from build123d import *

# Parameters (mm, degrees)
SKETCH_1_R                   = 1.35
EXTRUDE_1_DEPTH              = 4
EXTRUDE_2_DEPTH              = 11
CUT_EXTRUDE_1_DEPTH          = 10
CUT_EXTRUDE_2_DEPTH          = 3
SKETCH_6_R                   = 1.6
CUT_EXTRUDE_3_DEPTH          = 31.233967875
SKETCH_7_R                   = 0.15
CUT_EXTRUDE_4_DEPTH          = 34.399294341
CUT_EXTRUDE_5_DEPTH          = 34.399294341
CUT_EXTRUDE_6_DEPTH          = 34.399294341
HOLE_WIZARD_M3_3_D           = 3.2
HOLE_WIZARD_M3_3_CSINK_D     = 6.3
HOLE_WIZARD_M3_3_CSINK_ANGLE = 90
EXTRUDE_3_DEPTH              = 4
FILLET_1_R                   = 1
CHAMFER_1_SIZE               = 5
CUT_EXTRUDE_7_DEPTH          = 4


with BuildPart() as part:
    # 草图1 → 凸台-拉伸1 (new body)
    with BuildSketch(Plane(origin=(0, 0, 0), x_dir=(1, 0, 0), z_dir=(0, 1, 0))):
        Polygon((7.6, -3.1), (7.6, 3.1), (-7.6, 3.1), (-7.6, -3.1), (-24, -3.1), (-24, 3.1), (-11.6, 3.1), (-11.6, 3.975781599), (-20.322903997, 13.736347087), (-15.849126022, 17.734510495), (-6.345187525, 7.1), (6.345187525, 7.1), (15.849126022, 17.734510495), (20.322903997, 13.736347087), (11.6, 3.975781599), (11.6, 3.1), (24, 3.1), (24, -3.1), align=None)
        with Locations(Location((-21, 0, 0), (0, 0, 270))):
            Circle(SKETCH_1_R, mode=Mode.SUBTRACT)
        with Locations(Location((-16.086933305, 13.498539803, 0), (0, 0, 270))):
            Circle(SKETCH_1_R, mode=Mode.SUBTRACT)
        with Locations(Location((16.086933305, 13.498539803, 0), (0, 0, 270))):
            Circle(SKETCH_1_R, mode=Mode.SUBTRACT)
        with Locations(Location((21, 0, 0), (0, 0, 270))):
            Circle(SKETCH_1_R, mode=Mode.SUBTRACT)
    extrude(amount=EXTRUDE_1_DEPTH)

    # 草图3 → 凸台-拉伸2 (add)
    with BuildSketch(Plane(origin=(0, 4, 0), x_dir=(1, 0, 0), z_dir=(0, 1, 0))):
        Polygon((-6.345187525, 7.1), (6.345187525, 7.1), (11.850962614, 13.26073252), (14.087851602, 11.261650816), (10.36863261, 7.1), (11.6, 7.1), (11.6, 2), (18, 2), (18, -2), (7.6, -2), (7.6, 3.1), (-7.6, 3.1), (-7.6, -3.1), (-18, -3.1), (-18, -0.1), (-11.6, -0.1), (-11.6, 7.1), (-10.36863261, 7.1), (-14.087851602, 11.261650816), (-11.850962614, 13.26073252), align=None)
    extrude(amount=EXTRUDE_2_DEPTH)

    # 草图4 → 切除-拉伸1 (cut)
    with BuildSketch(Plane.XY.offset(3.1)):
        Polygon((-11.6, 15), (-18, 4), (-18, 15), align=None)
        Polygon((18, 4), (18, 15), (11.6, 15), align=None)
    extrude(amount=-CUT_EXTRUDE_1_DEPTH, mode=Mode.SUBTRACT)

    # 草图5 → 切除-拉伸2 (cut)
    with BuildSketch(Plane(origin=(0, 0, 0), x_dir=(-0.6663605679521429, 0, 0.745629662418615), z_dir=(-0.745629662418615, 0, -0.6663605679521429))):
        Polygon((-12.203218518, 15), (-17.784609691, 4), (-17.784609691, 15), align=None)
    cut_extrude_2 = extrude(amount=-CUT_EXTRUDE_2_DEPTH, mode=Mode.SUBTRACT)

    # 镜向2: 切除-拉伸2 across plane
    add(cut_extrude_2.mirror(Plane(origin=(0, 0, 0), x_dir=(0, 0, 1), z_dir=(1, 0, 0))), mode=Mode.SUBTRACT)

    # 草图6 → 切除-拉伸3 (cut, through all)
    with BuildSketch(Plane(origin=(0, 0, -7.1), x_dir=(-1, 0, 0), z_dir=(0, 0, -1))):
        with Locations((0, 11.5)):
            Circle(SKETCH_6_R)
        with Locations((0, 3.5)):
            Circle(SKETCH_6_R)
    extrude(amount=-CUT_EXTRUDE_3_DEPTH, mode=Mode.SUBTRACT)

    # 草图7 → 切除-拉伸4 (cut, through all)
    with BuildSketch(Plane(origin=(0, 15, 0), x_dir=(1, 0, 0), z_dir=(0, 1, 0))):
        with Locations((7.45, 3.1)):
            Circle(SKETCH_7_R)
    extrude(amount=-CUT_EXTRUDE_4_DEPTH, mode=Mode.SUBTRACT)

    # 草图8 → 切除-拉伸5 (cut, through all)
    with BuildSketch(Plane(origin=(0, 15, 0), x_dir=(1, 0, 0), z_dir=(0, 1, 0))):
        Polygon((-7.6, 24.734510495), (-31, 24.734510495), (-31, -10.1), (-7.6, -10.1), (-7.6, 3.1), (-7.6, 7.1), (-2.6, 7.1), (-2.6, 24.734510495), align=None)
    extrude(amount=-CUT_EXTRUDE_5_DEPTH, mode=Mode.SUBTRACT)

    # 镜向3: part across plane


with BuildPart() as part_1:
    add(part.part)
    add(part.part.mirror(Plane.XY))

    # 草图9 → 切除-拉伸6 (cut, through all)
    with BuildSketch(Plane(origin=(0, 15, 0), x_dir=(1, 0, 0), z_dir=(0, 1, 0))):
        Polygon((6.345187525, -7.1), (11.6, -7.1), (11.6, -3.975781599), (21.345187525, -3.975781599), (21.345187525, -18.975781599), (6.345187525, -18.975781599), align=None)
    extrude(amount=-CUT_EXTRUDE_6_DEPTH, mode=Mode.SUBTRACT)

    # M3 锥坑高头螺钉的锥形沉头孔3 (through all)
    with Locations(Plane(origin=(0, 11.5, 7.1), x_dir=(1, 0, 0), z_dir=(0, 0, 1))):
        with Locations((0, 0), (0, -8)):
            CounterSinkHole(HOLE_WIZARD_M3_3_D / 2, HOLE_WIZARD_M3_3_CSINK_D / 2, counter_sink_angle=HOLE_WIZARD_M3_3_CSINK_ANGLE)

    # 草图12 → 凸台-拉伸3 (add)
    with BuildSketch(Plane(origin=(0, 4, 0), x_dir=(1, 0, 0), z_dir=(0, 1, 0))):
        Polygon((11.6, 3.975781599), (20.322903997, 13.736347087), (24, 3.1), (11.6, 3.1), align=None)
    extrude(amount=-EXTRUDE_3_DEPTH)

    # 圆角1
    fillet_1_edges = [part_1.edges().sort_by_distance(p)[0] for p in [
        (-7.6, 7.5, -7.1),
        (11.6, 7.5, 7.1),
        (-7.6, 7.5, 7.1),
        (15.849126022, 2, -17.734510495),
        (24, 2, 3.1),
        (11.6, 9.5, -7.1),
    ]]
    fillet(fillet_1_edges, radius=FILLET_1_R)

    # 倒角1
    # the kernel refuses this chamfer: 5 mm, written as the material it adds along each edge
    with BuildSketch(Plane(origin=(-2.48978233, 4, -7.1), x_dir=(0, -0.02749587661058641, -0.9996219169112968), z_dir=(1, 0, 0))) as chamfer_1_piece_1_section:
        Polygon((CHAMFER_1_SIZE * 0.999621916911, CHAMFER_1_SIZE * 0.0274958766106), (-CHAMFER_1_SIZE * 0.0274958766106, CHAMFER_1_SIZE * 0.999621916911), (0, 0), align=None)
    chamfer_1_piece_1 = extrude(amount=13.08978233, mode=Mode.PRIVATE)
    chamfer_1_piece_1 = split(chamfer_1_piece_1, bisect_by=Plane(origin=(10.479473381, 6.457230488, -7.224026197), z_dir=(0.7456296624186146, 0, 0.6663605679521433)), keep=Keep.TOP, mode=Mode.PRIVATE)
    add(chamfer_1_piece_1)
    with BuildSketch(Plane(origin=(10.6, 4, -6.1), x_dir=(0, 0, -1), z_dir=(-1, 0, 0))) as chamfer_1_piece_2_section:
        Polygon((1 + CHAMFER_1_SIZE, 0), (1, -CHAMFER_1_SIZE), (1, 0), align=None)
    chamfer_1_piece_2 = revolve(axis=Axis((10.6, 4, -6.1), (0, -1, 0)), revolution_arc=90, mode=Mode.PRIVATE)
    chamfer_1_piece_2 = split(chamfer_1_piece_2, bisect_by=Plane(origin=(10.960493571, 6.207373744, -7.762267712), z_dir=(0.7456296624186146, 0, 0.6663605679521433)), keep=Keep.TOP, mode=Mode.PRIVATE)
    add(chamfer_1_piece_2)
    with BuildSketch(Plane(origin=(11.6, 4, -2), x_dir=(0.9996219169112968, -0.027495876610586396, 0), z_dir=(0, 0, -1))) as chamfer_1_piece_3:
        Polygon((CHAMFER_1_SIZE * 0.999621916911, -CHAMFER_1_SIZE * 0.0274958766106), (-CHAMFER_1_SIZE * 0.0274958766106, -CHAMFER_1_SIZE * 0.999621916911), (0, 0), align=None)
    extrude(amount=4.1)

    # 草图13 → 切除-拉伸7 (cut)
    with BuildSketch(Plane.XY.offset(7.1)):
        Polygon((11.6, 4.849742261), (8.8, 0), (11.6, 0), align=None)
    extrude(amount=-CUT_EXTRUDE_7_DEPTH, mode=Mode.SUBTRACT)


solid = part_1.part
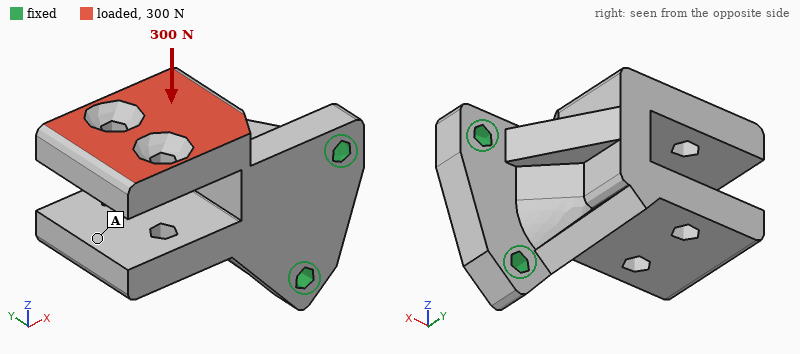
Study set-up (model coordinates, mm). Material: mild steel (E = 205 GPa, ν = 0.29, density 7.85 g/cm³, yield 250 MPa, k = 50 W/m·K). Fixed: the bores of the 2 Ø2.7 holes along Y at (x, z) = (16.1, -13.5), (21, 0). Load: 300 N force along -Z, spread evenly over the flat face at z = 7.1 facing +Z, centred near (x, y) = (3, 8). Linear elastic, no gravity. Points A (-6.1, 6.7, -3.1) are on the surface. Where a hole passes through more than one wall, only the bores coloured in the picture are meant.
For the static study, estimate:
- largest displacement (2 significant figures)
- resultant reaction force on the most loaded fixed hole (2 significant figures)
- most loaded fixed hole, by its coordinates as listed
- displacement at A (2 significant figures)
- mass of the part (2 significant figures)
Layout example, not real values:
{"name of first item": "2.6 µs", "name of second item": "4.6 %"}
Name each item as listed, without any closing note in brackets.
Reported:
{"largest displacement": "27 µm", "resultant reaction force on the most loaded fixed hole": "430 N", "most loaded fixed hole, by its coordinates as listed": "(16.1, -13.5)", "displacement at A": "4.5 µm", "mass of the part": "29 g"}
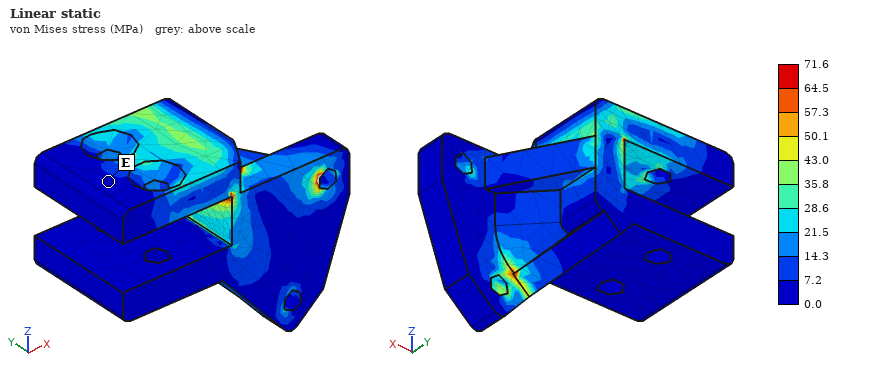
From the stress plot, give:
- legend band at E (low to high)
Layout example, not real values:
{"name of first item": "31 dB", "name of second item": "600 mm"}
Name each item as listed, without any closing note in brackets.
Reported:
{"legend band at E": "0.0 to 7.2 MPa"}
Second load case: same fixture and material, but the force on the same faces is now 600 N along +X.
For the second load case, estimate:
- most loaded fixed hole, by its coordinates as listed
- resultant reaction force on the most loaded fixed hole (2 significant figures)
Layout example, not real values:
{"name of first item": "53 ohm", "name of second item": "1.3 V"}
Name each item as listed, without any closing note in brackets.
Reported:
{"most loaded fixed hole, by its coordinates as listed": "(21, 0)", "resultant reaction force on the most loaded fixed hole": "860 N"}
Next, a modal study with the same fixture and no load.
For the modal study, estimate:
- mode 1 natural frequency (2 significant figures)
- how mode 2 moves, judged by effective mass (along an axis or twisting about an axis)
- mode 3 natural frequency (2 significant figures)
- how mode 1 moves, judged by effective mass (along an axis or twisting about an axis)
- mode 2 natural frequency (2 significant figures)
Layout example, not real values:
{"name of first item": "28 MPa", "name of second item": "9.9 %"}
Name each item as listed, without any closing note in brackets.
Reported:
{"mode 1 natural frequency": "3800 Hz", "how mode 2 moves, judged by effective mass": "along Z", "mode 3 natural frequency": "11 kHz", "how mode 1 moves, judged by effective mass": "along Y", "mode 2 natural frequency": "6800 Hz"}
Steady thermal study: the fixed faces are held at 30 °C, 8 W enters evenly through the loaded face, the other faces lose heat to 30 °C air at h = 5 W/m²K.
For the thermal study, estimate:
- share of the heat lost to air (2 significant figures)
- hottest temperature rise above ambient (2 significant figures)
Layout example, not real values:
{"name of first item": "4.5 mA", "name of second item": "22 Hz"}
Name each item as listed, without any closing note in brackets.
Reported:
{"share of the heat lost to air": "3.4 %", "hottest temperature rise above ambient": "56 K"}
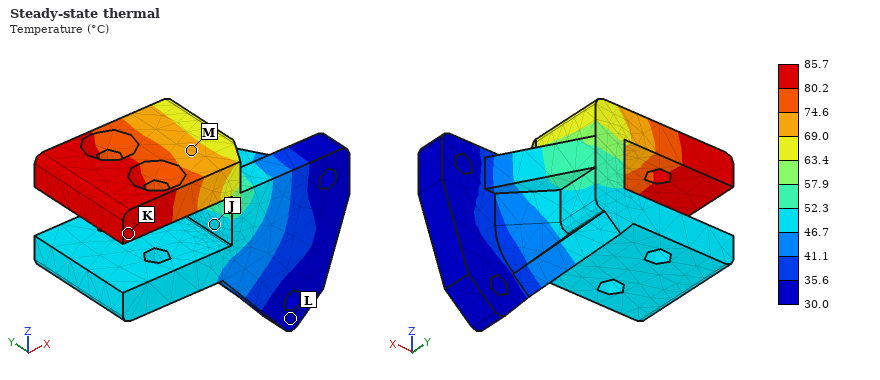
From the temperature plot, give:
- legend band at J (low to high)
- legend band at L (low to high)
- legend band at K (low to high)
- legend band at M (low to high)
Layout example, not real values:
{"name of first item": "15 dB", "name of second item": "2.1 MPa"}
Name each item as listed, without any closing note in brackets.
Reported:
{"legend band at J": "46.7 to 52.3 °C", "legend band at L": "30.0 to 35.6 °C", "legend band at K": "80.2 to 85.7 °C", "legend band at M": "69.0 to 74.6 °C"}
